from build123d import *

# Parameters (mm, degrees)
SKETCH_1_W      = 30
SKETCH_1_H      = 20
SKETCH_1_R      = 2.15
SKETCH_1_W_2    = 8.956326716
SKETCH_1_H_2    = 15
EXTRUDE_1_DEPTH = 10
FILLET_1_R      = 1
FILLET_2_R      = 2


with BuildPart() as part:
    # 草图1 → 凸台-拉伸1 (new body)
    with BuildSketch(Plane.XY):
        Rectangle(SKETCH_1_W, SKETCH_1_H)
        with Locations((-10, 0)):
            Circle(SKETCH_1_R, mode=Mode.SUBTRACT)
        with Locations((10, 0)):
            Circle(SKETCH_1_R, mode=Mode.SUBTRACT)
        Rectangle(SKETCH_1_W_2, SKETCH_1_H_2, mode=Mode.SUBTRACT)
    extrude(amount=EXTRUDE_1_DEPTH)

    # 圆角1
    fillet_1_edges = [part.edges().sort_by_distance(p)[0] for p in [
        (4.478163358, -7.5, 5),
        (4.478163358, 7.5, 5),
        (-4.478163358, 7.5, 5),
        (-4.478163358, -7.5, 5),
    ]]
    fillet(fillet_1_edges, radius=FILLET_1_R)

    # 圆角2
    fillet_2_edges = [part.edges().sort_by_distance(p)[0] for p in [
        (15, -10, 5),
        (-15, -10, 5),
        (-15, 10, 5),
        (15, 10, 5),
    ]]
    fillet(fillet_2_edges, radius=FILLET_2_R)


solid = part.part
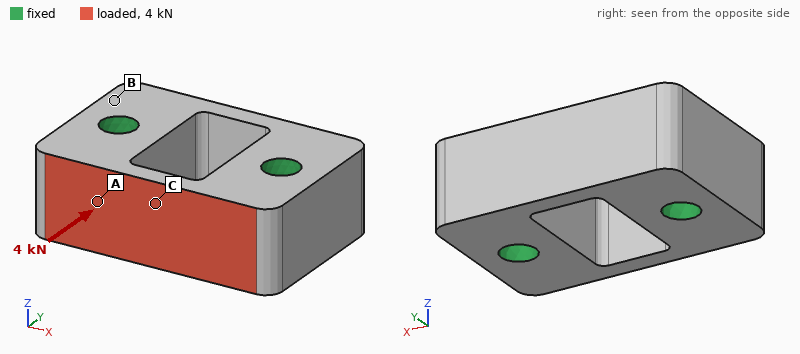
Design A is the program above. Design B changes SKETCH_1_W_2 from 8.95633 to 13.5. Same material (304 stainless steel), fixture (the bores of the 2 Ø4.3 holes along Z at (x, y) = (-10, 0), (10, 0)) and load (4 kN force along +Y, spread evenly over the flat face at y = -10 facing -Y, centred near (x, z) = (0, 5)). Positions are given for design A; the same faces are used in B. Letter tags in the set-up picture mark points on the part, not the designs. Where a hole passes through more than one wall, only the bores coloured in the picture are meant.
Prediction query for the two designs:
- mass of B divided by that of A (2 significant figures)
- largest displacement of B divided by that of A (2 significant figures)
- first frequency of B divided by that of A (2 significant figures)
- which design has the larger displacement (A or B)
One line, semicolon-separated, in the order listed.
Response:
0.84; 2.7; 0.94; B
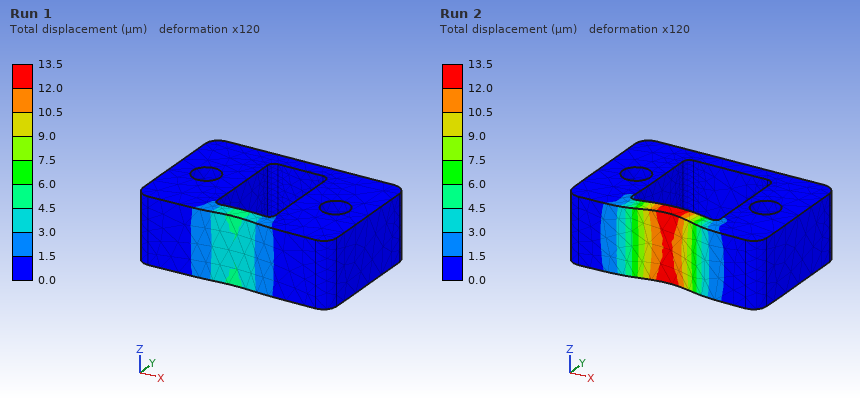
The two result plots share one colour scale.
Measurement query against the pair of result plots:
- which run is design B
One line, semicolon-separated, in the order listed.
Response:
Run 2
